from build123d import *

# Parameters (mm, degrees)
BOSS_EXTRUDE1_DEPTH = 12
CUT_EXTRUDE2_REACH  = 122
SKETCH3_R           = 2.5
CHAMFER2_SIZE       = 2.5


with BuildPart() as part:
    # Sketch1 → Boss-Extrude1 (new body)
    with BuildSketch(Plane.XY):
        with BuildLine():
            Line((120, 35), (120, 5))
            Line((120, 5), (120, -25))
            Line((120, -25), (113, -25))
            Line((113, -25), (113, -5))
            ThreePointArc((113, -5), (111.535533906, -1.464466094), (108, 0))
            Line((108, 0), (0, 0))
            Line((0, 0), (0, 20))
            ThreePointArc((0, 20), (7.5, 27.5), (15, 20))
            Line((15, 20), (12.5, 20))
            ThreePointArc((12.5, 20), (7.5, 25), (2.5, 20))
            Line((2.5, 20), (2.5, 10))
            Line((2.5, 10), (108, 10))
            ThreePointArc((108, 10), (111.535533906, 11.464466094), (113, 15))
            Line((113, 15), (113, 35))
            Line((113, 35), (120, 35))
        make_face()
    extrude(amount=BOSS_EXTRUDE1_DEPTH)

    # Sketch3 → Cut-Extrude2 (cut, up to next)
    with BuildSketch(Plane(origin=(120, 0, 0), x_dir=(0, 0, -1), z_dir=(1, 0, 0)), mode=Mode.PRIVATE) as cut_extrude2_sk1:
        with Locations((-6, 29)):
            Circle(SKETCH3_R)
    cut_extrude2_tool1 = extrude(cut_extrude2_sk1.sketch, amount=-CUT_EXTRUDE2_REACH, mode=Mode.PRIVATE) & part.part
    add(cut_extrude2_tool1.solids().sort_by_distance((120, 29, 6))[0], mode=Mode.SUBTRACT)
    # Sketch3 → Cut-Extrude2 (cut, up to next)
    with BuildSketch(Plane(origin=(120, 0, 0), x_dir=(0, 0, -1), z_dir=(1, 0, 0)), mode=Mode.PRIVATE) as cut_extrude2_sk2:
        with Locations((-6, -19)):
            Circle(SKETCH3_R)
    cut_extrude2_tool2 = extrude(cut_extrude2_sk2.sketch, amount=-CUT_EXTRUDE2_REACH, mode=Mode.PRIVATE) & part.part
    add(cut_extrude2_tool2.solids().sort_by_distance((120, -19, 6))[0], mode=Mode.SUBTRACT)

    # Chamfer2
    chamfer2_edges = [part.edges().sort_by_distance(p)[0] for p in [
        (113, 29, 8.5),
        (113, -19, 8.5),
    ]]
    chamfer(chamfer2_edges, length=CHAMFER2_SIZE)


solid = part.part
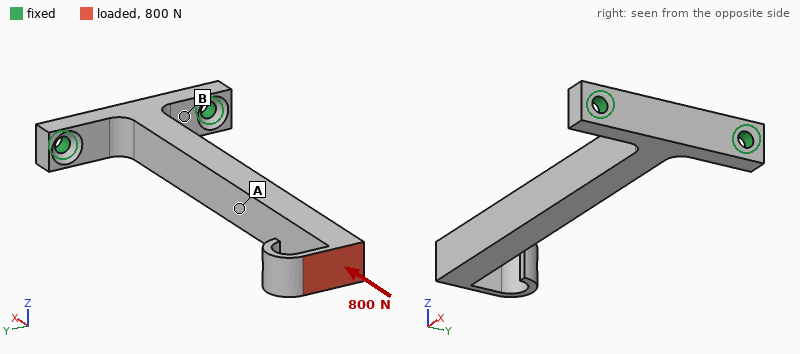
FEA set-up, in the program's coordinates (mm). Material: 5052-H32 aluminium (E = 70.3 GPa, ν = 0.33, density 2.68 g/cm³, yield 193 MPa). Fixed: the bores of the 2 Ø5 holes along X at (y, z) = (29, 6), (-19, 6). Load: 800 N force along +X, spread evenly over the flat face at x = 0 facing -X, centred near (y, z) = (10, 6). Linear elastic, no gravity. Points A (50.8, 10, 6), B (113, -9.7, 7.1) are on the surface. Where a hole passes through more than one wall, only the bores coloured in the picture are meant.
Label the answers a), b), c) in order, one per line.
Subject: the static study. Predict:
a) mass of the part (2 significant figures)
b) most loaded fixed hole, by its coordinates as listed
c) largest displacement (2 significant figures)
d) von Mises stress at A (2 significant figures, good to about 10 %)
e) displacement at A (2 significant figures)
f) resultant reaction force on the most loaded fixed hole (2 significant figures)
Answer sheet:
a) 51 g
b) (29, 6)
c) 0.46 mm
d) 27 MPa
e) 0.13 mm
f) 610 N
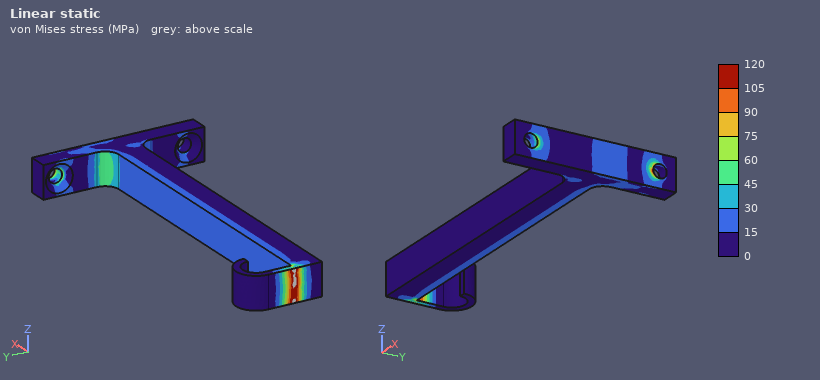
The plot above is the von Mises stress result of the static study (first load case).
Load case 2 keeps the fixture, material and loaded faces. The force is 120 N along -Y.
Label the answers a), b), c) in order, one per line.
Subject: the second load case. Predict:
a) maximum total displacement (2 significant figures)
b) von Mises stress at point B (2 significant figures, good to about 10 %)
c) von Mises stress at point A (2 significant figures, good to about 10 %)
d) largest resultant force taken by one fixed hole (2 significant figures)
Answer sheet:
a) 0.95 mm
b) 14 MPa
c) 30 MPa
d) 400 N
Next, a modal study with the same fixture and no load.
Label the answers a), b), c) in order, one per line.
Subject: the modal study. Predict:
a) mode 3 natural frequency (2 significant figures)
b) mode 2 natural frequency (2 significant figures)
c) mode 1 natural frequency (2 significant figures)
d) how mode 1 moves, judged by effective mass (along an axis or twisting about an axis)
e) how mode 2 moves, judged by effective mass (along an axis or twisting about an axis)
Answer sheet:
a) 2800 Hz
b) 540 Hz
c) 430 Hz
d) along Z
e) along Y
